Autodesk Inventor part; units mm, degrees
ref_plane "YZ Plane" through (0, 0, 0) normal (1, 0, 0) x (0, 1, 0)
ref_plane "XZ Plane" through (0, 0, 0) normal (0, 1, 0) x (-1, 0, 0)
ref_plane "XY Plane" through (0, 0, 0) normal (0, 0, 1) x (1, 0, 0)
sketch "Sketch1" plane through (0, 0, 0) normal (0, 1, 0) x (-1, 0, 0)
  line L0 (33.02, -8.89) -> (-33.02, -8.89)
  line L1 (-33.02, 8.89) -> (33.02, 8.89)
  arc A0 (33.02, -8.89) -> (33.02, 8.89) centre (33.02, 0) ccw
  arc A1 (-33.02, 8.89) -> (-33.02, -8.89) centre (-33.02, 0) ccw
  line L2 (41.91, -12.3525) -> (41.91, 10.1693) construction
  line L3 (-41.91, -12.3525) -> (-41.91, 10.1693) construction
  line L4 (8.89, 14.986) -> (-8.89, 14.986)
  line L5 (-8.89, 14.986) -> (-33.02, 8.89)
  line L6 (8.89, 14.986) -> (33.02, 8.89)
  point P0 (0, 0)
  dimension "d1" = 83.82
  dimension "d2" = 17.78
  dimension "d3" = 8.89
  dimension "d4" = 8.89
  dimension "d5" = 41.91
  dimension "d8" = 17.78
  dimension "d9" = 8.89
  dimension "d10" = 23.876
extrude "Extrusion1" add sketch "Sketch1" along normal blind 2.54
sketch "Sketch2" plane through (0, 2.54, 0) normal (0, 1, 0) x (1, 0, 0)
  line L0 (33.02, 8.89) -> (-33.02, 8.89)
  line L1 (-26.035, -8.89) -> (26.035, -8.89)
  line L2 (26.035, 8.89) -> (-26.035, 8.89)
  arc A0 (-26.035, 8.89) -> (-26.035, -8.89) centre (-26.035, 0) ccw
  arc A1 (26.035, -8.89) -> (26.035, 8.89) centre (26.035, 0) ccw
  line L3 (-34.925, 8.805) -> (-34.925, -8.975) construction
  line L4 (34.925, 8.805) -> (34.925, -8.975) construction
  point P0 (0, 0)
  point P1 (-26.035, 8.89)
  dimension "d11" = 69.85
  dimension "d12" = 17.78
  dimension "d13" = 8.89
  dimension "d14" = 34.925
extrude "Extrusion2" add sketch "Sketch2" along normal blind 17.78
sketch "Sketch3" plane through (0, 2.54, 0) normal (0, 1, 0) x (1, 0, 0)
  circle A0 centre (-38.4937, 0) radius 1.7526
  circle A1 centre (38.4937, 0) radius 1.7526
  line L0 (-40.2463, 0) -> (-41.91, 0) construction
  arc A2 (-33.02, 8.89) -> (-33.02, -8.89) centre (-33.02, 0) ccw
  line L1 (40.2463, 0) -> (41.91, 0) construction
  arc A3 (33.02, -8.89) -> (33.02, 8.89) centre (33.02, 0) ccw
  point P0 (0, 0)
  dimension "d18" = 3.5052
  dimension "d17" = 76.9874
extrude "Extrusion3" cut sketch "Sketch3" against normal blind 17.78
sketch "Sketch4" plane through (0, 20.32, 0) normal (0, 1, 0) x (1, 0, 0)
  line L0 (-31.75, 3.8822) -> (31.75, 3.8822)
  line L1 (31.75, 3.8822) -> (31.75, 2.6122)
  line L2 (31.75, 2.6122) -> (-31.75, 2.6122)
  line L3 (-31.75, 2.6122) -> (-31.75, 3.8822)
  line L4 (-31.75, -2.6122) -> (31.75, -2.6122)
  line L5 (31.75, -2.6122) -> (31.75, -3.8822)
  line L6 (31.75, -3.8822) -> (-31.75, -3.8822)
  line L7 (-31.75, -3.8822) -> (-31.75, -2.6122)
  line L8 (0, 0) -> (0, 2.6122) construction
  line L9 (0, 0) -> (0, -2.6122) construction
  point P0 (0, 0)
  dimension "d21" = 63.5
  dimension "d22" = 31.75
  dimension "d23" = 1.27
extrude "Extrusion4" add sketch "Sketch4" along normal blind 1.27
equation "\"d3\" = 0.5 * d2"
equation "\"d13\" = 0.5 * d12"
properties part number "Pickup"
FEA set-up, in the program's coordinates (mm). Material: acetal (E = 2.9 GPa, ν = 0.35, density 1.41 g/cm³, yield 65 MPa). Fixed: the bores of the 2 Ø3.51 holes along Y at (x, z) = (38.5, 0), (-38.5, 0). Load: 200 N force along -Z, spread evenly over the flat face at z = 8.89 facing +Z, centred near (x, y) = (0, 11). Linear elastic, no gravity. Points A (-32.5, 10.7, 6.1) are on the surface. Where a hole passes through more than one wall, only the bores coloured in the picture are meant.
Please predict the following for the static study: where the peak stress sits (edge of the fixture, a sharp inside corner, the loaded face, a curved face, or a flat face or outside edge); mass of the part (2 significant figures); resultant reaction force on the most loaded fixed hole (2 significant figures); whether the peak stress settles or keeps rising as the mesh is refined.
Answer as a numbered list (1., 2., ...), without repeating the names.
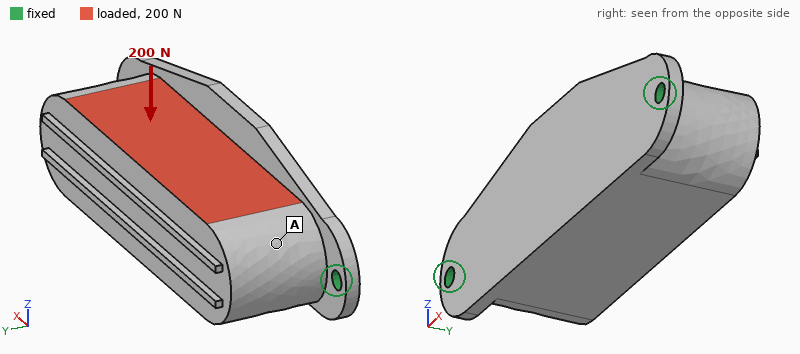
1. edge of the fixture
2. 36 g
3. 100 N
4. keeps rising
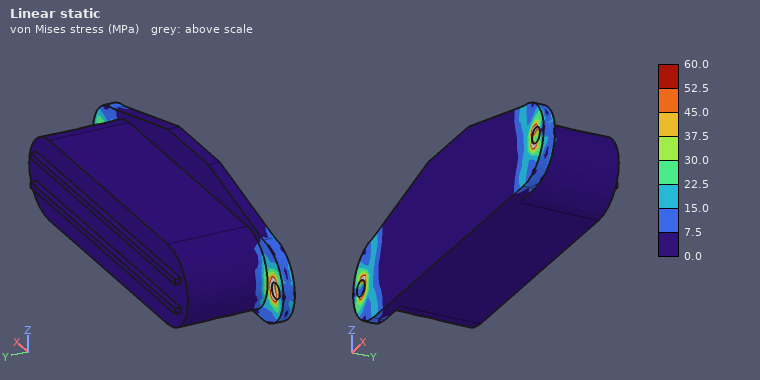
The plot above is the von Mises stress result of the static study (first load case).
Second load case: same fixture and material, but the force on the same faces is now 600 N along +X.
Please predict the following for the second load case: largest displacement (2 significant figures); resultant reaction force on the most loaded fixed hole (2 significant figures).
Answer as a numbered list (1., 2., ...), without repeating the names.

1. 63 µm
2. 320 N
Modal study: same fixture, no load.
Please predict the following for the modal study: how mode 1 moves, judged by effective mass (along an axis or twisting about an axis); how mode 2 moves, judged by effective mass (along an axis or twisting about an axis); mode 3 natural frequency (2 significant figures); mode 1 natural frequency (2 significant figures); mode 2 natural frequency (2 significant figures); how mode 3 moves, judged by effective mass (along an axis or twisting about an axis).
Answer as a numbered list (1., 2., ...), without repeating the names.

1. along Z
2. along Y
3. 2400 Hz
4. 490 Hz
5. 1700 Hz
6. along Z
